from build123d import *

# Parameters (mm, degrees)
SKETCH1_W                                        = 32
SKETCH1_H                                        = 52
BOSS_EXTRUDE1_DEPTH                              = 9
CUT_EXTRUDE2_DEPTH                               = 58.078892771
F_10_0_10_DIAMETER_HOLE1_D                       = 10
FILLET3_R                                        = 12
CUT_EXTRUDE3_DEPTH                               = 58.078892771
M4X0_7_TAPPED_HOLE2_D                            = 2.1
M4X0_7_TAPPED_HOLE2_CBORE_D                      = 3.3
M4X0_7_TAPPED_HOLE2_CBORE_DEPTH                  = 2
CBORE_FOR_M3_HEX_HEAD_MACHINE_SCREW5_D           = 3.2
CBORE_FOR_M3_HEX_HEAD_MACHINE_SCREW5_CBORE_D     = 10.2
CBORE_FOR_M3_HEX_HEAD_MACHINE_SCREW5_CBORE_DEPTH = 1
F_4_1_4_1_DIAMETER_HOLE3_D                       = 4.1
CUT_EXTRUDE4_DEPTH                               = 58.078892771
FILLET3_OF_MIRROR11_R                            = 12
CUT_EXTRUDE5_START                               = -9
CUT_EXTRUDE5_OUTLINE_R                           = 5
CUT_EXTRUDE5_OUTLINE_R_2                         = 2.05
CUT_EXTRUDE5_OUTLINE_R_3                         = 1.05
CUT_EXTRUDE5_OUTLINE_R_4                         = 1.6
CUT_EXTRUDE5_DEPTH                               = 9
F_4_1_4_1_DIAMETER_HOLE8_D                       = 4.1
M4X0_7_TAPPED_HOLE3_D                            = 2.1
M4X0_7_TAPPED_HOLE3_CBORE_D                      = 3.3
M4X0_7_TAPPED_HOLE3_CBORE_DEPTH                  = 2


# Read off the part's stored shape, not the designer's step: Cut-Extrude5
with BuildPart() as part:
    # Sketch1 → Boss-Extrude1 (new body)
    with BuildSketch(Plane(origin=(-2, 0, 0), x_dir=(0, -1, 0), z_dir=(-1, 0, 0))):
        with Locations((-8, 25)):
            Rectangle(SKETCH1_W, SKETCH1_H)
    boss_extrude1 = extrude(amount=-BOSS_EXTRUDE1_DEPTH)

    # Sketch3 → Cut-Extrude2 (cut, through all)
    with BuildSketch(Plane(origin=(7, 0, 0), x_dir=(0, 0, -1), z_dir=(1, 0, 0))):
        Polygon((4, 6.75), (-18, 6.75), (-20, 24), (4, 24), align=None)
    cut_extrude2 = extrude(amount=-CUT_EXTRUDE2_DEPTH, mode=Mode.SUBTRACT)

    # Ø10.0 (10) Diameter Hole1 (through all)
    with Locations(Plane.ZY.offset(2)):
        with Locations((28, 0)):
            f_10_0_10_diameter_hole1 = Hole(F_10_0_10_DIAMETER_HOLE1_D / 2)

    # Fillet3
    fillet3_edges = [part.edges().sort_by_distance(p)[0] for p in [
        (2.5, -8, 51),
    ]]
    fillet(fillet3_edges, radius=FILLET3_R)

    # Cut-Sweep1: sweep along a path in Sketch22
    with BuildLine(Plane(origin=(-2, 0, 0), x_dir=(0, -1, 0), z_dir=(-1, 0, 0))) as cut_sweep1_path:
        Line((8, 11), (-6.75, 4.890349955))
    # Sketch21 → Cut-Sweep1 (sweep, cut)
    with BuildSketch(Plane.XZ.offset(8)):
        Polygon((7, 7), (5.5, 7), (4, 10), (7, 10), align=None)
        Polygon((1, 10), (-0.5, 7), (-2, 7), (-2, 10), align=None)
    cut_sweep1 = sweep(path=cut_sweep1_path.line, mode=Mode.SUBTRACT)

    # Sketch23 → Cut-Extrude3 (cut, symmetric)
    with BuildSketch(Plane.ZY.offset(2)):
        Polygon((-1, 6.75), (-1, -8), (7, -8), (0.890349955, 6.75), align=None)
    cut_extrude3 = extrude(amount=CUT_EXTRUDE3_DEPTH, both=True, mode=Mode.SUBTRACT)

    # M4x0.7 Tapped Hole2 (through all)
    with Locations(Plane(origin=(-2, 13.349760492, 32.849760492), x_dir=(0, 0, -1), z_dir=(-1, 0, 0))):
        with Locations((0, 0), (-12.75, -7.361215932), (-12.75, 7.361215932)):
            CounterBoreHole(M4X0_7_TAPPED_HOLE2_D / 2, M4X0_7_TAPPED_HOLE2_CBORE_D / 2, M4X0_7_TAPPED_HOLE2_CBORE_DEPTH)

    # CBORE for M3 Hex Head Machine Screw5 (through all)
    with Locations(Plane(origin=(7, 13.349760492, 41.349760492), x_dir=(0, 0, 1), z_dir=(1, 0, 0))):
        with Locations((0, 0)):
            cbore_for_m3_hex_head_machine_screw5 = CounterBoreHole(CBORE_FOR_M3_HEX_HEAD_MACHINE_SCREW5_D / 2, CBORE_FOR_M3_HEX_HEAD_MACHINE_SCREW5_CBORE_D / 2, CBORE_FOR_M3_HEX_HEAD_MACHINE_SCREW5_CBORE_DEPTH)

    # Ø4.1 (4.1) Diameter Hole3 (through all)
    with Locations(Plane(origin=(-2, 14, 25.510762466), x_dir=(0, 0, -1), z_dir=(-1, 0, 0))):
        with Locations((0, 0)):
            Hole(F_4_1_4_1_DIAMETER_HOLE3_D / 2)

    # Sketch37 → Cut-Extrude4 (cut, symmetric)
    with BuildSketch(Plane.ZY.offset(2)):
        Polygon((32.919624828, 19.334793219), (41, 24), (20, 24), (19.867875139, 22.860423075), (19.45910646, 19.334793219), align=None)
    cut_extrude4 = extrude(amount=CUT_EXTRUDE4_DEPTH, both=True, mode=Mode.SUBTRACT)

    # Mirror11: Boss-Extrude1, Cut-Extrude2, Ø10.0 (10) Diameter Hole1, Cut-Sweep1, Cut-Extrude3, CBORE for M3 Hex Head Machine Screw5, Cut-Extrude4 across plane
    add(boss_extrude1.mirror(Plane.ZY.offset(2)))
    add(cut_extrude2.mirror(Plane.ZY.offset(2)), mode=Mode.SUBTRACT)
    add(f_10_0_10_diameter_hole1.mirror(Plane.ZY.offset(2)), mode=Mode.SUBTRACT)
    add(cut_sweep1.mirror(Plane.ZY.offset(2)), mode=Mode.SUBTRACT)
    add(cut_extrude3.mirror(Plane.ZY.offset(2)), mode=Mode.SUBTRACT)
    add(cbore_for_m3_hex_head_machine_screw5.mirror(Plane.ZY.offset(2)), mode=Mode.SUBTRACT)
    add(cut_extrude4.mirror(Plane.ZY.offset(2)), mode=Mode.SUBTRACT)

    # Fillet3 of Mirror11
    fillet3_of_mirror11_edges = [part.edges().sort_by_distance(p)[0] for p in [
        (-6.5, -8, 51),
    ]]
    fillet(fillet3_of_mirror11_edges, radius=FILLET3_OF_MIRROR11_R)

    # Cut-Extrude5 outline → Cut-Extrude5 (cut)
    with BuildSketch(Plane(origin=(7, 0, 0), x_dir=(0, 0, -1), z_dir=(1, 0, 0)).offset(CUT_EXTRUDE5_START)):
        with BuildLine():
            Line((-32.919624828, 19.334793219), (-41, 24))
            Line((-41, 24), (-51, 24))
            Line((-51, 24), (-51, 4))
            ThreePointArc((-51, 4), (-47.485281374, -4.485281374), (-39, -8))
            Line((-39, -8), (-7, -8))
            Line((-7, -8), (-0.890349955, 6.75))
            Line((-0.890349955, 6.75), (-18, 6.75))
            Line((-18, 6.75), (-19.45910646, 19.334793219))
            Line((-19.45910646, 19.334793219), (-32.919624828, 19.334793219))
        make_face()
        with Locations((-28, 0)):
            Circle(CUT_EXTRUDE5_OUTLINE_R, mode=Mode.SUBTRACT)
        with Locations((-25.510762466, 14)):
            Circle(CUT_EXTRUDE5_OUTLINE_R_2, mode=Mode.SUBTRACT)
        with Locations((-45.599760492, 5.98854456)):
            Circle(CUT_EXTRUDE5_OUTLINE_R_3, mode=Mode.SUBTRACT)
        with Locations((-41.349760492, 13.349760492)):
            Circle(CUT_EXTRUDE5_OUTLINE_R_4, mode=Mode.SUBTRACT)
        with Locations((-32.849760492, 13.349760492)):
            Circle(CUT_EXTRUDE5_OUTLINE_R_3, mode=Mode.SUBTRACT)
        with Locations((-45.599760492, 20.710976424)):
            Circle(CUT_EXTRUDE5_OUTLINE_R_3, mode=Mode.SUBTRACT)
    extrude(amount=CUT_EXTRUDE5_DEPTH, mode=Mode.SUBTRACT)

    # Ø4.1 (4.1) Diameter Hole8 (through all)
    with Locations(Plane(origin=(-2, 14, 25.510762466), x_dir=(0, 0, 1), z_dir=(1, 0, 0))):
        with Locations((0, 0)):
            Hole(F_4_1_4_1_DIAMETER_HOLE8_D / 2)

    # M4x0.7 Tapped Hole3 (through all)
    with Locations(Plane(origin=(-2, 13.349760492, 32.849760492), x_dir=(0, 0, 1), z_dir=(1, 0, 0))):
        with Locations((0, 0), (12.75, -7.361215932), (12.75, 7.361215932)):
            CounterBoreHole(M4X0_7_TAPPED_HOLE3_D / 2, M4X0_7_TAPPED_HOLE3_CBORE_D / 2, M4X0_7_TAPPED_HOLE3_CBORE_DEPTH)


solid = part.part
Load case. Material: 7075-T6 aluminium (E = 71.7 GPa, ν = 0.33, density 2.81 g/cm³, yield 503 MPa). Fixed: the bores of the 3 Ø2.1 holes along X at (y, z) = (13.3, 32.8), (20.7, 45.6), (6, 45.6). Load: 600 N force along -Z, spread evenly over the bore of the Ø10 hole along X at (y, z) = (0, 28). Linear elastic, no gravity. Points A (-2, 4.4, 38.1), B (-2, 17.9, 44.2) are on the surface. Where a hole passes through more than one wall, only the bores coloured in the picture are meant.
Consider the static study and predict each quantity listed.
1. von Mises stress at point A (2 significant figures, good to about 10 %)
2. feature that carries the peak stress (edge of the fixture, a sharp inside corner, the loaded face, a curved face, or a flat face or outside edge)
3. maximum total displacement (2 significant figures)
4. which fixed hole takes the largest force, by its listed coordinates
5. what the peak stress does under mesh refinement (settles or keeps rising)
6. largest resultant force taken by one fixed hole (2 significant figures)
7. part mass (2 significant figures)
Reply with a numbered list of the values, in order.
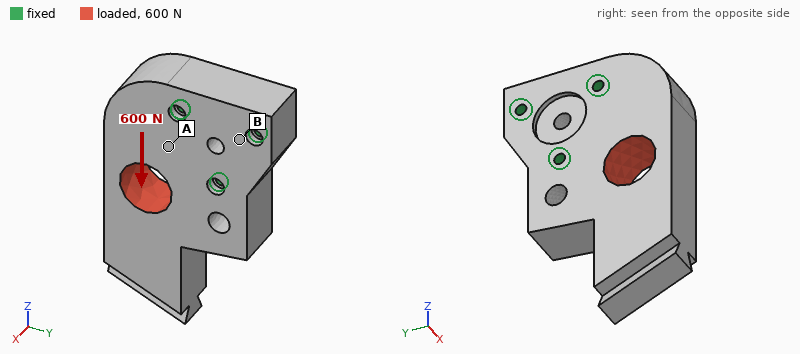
1. 4.8 MPa
2. edge of the fixture
3. 5.6 µm
4. (6, 45.6)
5. keeps rising
6. 520 N
7. 25 g
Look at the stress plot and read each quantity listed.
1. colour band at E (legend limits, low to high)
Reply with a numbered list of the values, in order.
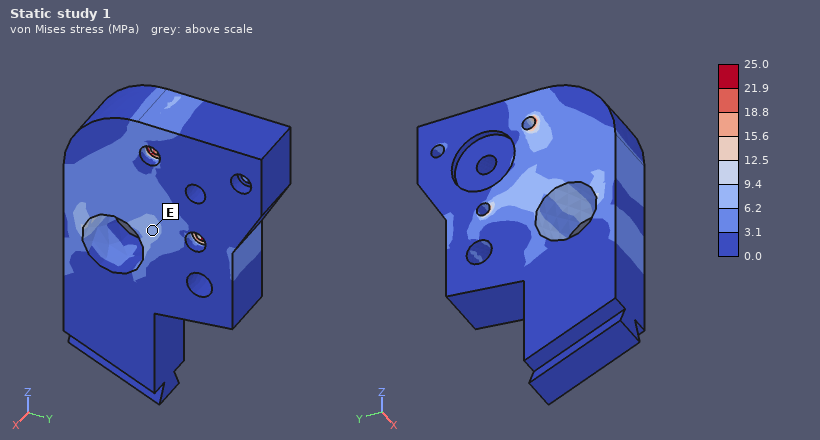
1. 6.2 to 9.4 MPa
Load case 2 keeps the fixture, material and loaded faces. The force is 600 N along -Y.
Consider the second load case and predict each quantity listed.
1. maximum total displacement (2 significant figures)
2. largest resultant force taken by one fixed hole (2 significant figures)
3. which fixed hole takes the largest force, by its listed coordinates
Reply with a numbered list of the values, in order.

1. 4.7 µm
2. 620 N
3. (13.3, 32.8)
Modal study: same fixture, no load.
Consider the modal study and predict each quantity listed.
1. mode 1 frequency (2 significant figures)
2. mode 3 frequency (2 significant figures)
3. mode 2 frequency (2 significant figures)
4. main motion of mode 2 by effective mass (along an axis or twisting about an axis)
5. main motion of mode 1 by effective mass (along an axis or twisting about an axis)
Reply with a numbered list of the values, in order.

1. 5800 Hz
2. 15 kHz
3. 12 kHz
4. along Y
5. along X
